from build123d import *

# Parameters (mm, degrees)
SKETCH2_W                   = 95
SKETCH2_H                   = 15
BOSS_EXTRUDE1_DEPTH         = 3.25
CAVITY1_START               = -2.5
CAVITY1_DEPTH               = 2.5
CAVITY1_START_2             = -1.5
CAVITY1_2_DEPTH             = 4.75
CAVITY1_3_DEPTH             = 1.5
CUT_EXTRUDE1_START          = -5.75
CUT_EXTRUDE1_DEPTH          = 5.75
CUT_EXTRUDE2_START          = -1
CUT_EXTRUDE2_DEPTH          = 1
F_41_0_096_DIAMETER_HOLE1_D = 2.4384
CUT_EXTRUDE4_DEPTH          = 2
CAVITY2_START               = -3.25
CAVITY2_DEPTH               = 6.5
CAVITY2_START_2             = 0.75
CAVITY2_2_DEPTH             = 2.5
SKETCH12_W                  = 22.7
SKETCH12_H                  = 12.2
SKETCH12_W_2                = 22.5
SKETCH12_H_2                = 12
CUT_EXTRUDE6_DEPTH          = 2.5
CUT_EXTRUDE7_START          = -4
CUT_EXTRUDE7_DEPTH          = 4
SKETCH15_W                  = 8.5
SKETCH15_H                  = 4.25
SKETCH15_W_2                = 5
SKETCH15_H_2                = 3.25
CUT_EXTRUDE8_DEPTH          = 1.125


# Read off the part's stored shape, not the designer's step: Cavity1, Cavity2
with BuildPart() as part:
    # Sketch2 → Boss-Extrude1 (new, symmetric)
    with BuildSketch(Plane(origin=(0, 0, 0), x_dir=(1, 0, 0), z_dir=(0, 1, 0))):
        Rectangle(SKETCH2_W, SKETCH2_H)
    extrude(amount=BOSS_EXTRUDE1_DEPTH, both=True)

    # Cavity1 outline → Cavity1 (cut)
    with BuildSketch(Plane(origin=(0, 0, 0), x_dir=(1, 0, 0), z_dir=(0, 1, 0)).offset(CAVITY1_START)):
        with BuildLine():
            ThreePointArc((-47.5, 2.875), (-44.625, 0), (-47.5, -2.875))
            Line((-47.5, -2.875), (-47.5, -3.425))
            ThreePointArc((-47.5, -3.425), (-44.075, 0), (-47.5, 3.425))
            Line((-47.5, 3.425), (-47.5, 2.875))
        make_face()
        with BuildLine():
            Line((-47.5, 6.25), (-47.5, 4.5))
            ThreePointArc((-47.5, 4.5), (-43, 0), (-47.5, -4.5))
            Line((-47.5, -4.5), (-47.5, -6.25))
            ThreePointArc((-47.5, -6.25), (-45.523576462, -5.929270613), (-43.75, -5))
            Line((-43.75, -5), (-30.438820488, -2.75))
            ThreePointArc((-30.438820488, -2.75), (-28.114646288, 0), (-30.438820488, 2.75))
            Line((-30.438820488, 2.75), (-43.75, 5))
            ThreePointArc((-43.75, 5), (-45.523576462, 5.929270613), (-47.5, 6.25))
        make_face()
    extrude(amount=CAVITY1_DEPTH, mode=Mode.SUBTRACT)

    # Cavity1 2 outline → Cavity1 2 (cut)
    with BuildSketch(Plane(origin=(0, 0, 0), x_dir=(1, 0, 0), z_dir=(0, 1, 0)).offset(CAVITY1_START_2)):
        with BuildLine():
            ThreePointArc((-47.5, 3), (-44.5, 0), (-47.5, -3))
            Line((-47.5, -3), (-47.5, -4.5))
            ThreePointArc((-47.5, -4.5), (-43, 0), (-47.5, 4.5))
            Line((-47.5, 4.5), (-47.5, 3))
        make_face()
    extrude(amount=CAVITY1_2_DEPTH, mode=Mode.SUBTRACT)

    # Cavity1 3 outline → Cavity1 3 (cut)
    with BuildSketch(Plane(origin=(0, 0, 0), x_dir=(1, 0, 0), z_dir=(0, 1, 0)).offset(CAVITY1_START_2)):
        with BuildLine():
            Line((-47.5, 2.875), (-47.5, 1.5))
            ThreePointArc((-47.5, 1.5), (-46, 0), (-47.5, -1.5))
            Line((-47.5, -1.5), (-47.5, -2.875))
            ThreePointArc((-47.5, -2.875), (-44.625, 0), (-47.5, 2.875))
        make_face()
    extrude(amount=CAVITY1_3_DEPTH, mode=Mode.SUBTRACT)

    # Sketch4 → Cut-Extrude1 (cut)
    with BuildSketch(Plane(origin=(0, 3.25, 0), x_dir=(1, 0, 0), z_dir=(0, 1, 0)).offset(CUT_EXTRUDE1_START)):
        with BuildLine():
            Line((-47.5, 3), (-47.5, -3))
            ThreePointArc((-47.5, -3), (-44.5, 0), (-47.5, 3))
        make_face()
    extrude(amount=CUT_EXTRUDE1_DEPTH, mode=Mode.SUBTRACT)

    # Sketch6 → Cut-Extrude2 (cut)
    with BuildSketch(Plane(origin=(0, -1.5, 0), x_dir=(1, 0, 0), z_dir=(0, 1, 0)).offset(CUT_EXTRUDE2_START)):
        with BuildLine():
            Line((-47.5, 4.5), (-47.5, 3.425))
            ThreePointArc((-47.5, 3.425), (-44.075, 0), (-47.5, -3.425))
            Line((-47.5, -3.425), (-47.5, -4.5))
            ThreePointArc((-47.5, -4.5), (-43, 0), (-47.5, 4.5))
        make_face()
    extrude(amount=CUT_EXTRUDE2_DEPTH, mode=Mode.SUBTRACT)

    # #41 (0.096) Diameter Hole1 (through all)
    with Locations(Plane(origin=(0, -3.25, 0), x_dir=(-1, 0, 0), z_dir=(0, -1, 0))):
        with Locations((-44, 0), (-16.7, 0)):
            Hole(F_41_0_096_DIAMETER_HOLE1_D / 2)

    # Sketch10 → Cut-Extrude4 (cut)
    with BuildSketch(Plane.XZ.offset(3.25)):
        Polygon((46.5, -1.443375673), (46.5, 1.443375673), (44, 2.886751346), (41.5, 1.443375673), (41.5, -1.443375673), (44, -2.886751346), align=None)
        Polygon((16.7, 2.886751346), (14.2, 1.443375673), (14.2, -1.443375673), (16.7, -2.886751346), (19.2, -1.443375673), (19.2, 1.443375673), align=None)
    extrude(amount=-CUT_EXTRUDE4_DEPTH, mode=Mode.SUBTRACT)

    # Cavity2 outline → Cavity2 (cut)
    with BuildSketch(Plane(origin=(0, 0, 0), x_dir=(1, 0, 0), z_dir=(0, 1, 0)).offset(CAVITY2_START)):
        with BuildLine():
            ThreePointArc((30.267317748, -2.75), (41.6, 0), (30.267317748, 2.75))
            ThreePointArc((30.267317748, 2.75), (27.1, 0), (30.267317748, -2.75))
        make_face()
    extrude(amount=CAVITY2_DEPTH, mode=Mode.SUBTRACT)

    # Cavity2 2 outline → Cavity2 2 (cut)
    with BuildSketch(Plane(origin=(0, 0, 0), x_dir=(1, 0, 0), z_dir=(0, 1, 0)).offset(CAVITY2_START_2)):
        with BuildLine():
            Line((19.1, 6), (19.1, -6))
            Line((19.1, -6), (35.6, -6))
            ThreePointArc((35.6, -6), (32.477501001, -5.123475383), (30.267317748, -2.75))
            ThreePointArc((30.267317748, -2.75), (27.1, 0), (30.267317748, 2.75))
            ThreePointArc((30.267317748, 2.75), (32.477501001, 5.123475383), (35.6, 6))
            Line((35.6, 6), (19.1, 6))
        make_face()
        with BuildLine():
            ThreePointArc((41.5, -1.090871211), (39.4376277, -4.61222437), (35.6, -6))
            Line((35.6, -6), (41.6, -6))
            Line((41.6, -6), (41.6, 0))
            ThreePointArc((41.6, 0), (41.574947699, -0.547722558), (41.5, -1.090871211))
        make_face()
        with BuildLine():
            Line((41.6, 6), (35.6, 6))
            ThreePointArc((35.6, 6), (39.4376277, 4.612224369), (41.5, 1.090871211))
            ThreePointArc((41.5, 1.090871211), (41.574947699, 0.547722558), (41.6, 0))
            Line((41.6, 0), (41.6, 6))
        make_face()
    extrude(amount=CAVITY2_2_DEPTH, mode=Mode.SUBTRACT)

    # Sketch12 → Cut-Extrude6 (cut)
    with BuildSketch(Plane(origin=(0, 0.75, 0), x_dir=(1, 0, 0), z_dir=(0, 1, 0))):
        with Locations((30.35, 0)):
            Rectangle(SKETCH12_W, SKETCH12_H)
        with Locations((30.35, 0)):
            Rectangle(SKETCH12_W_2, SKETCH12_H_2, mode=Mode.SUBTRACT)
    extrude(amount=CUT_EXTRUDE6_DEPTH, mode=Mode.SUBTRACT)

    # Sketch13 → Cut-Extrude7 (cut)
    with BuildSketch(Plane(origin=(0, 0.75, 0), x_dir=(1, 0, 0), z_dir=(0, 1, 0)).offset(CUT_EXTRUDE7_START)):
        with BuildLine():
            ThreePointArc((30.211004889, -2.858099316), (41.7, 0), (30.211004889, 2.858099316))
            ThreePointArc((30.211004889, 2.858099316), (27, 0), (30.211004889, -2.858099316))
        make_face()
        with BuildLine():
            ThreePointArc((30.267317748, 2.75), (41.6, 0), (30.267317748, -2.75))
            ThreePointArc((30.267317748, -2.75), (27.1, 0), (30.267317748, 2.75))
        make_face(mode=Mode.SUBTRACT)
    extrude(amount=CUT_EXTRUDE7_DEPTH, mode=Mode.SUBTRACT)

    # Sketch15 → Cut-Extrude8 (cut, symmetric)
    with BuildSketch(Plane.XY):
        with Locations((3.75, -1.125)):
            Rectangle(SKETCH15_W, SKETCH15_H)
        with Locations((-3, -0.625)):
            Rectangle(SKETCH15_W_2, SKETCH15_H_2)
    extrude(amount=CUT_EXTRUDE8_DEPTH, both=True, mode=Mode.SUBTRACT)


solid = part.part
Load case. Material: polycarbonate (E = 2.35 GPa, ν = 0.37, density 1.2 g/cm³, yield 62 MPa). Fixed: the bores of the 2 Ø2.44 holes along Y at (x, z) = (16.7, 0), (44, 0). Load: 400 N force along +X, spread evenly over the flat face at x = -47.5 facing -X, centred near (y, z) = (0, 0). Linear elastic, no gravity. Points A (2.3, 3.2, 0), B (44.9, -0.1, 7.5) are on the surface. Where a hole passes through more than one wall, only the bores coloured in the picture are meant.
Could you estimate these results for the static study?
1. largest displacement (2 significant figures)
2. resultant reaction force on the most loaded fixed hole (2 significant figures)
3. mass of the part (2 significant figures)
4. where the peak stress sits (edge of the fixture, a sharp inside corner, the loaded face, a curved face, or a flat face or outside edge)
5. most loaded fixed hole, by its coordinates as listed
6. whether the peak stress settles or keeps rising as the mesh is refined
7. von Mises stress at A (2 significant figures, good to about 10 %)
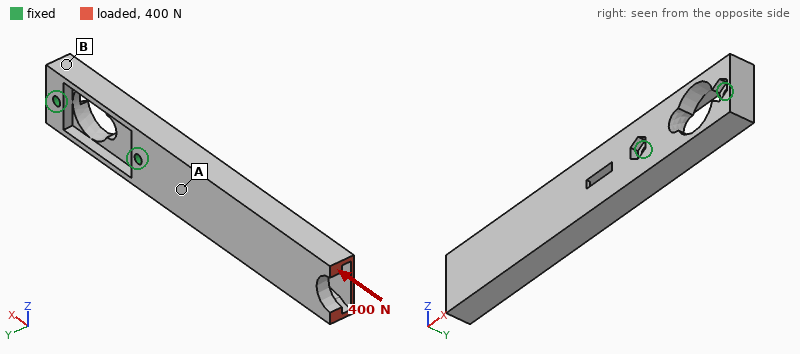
0.59 mm
370 N
8.8 g
edge of the fixture
(16.7, 0)
keeps rising
3.7 MPa
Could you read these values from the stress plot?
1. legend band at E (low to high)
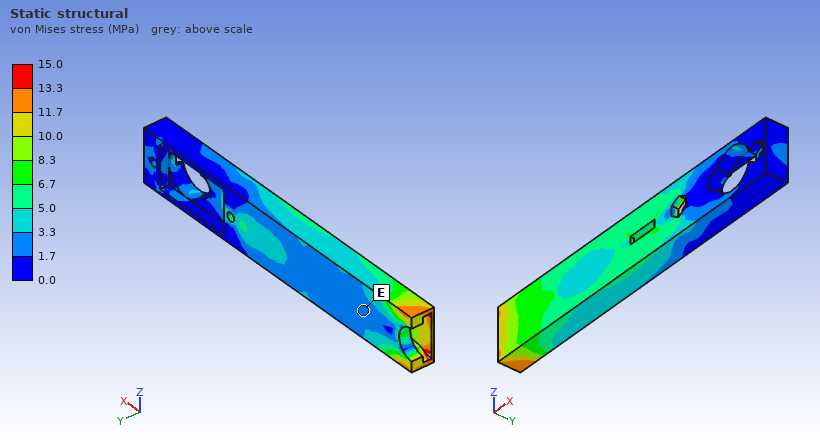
1.7 to 3.3 MPa
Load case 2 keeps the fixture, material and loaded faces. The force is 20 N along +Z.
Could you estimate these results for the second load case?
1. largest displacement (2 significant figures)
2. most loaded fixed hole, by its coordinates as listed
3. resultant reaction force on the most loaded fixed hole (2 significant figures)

0.94 mm
(16.7, 0)
40 N
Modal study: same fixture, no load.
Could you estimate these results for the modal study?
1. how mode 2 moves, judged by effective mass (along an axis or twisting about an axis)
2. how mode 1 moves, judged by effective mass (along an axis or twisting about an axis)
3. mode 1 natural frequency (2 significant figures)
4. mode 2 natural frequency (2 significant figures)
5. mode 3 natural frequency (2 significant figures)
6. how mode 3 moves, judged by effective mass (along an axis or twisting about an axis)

along Z
along Y
340 Hz
560 Hz
2000 Hz
twisting about X
